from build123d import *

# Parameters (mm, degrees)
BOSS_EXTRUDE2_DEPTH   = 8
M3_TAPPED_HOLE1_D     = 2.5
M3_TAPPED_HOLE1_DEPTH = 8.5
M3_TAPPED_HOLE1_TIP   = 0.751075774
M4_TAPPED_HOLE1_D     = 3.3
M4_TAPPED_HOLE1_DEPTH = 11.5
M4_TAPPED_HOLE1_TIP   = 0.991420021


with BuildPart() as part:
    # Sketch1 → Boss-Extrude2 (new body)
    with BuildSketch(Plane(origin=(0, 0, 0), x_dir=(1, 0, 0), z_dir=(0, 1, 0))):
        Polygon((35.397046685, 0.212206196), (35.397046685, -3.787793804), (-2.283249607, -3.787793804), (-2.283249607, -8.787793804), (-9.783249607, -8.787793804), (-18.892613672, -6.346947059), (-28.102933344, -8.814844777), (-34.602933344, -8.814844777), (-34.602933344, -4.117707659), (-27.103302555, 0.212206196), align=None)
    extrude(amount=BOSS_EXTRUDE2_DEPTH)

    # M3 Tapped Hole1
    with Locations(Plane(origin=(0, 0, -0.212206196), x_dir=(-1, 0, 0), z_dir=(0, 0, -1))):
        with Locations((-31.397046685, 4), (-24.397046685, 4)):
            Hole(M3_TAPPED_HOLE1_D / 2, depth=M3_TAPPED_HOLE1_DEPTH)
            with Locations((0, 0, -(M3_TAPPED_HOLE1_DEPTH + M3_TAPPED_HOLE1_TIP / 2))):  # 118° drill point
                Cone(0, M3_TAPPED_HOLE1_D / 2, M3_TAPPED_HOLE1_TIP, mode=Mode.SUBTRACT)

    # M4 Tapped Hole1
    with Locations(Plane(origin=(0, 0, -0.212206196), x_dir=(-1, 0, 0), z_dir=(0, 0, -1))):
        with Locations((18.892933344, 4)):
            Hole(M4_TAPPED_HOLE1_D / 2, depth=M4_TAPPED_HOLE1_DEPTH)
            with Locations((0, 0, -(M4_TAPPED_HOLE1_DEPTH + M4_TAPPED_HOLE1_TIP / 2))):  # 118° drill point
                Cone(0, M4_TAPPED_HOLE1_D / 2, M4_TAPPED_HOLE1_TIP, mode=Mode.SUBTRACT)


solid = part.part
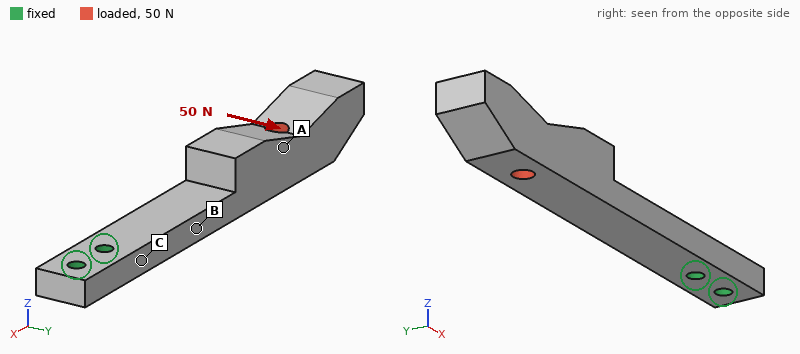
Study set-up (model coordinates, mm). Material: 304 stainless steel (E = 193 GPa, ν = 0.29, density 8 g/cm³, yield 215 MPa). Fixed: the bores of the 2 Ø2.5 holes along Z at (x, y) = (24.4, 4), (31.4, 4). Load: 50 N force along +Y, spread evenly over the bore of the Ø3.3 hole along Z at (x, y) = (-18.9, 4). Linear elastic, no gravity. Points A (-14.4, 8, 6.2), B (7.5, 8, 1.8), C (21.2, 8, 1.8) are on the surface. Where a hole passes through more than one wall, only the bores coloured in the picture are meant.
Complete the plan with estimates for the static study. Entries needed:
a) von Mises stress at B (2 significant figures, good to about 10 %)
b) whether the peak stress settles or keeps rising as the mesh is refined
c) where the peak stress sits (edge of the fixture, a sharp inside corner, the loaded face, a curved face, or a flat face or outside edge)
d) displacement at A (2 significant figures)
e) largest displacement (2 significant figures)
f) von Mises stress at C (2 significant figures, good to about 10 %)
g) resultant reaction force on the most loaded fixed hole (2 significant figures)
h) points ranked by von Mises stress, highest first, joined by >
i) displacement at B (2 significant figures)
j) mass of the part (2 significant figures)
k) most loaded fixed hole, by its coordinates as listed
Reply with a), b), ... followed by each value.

a) 31 MPa
b) keeps rising
c) edge of the fixture
d) 42 µm
e) 72 µm
f) 47 MPa
g) 200 N
h) C > B > A
i) 12 µm
j) 25 g
k) (24.4, 4)
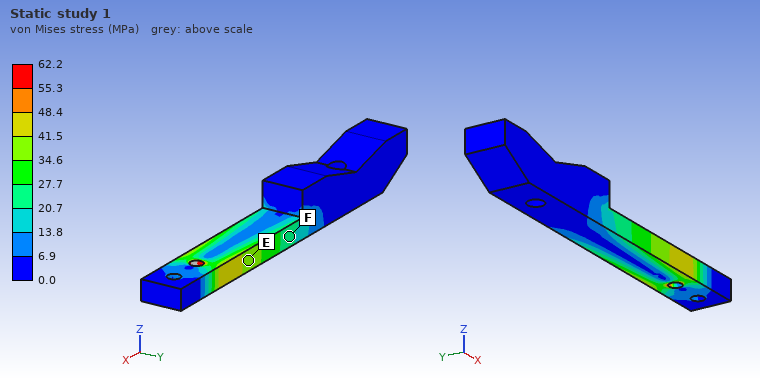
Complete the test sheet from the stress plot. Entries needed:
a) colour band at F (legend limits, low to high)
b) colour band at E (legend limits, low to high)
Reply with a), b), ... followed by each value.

a) 20.7 to 27.7 MPa
b) 34.6 to 41.5 MPa
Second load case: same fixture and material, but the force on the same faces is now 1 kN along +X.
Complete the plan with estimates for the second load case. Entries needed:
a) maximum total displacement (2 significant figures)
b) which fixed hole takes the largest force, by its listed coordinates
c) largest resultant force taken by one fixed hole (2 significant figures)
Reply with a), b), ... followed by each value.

a) 0.22 mm
b) (24.4, 4)
c) 880 N
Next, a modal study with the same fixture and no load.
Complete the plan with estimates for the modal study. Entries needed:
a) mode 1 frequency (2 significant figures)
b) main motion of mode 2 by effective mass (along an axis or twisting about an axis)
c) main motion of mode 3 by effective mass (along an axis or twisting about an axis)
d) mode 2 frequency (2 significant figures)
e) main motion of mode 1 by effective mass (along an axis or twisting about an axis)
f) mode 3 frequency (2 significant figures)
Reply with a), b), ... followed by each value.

a) 710 Hz
b) along Y
c) along Z
d) 1300 Hz
e) along Z
f) 5900 Hz
